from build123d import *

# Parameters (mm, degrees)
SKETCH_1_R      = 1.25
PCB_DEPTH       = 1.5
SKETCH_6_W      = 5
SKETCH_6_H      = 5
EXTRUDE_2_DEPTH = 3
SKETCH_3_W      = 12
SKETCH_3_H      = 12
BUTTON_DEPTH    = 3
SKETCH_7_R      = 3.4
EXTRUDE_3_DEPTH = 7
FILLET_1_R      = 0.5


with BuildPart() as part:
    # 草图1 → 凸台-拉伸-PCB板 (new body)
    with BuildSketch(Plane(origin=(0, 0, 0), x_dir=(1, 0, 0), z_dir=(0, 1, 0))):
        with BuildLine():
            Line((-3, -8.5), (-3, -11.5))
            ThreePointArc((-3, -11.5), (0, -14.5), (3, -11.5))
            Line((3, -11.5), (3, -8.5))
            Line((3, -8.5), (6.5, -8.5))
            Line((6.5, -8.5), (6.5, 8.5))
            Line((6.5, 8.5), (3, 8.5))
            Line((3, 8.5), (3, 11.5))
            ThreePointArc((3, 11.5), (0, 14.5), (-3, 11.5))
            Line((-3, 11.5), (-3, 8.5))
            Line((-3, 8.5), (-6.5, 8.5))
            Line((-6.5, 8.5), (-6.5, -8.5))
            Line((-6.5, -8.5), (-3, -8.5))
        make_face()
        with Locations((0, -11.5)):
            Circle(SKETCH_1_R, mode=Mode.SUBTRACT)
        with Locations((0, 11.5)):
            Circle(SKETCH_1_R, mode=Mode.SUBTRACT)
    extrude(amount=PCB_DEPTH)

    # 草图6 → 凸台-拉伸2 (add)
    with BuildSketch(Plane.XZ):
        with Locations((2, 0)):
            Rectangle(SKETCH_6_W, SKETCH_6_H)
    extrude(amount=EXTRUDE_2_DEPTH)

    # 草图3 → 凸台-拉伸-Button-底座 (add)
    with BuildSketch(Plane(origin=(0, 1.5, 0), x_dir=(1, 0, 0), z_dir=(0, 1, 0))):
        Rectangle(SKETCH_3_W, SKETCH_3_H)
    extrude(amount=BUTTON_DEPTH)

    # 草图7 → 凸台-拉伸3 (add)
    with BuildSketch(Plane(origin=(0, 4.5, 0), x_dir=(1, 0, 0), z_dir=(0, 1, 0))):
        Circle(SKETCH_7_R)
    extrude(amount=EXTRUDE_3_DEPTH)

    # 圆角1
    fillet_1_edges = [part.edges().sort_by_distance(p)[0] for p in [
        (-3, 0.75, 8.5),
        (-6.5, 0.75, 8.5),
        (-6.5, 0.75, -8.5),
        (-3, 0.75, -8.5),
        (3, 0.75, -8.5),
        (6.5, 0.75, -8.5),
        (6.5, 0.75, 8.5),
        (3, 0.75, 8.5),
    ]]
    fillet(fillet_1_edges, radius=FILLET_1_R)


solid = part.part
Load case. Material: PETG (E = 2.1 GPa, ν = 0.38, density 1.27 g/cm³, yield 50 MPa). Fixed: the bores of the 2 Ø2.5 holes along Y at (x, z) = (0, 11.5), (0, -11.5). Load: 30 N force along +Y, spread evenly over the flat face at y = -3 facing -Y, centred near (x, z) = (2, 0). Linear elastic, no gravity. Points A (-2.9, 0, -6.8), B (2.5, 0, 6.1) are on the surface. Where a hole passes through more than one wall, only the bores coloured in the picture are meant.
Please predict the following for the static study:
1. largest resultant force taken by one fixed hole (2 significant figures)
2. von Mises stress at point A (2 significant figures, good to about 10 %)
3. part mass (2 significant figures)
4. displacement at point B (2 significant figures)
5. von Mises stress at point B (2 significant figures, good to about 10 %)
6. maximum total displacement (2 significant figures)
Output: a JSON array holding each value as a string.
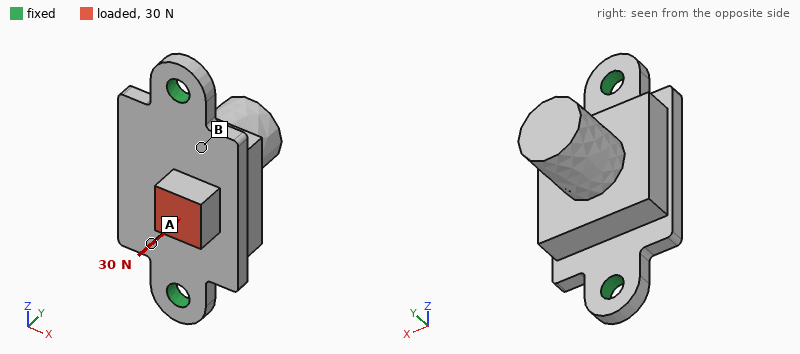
["17 N", "3.7 MPa", "1.5 g", "0.096 mm", "8.4 MPa", "0.24 mm"]
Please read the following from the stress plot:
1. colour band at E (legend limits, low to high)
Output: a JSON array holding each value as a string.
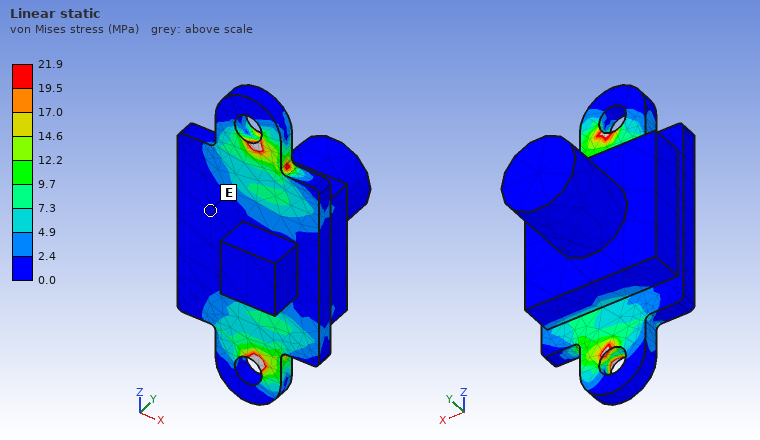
["0.0 to 2.4 MPa"]
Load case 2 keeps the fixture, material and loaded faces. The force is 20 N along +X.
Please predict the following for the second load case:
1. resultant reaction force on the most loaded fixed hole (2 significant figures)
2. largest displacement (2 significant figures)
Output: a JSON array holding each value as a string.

["10 N", "0.25 mm"]
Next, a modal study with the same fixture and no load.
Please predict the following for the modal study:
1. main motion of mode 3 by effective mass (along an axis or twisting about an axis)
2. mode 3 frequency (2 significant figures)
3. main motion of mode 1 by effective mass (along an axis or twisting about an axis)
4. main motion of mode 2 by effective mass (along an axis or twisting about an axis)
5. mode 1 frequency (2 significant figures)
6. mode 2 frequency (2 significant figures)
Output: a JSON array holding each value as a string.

["along Z", "5000 Hz", "along X", "along Y", "1500 Hz", "3100 Hz"]
